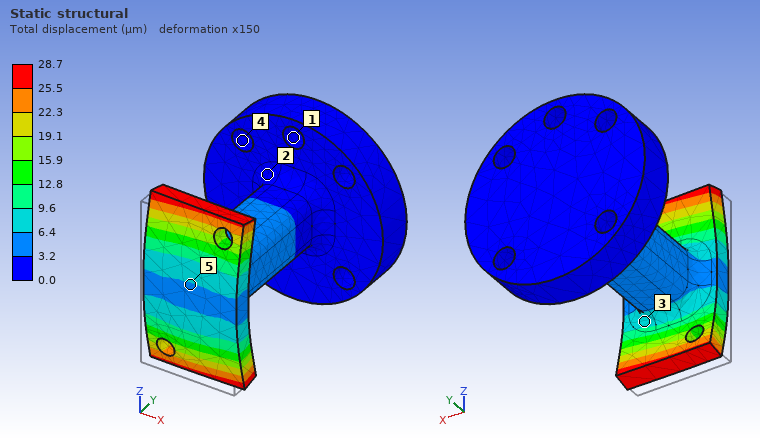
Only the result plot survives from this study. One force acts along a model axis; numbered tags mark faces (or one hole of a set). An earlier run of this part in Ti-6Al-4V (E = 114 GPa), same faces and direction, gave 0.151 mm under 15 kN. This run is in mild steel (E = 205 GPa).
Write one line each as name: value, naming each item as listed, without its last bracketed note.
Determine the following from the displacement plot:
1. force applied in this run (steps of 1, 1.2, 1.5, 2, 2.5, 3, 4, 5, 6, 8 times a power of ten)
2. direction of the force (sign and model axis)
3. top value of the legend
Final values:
force applied in this run: 5 kN
direction of the force: +Y
top value of the legend: 28.7 µm
